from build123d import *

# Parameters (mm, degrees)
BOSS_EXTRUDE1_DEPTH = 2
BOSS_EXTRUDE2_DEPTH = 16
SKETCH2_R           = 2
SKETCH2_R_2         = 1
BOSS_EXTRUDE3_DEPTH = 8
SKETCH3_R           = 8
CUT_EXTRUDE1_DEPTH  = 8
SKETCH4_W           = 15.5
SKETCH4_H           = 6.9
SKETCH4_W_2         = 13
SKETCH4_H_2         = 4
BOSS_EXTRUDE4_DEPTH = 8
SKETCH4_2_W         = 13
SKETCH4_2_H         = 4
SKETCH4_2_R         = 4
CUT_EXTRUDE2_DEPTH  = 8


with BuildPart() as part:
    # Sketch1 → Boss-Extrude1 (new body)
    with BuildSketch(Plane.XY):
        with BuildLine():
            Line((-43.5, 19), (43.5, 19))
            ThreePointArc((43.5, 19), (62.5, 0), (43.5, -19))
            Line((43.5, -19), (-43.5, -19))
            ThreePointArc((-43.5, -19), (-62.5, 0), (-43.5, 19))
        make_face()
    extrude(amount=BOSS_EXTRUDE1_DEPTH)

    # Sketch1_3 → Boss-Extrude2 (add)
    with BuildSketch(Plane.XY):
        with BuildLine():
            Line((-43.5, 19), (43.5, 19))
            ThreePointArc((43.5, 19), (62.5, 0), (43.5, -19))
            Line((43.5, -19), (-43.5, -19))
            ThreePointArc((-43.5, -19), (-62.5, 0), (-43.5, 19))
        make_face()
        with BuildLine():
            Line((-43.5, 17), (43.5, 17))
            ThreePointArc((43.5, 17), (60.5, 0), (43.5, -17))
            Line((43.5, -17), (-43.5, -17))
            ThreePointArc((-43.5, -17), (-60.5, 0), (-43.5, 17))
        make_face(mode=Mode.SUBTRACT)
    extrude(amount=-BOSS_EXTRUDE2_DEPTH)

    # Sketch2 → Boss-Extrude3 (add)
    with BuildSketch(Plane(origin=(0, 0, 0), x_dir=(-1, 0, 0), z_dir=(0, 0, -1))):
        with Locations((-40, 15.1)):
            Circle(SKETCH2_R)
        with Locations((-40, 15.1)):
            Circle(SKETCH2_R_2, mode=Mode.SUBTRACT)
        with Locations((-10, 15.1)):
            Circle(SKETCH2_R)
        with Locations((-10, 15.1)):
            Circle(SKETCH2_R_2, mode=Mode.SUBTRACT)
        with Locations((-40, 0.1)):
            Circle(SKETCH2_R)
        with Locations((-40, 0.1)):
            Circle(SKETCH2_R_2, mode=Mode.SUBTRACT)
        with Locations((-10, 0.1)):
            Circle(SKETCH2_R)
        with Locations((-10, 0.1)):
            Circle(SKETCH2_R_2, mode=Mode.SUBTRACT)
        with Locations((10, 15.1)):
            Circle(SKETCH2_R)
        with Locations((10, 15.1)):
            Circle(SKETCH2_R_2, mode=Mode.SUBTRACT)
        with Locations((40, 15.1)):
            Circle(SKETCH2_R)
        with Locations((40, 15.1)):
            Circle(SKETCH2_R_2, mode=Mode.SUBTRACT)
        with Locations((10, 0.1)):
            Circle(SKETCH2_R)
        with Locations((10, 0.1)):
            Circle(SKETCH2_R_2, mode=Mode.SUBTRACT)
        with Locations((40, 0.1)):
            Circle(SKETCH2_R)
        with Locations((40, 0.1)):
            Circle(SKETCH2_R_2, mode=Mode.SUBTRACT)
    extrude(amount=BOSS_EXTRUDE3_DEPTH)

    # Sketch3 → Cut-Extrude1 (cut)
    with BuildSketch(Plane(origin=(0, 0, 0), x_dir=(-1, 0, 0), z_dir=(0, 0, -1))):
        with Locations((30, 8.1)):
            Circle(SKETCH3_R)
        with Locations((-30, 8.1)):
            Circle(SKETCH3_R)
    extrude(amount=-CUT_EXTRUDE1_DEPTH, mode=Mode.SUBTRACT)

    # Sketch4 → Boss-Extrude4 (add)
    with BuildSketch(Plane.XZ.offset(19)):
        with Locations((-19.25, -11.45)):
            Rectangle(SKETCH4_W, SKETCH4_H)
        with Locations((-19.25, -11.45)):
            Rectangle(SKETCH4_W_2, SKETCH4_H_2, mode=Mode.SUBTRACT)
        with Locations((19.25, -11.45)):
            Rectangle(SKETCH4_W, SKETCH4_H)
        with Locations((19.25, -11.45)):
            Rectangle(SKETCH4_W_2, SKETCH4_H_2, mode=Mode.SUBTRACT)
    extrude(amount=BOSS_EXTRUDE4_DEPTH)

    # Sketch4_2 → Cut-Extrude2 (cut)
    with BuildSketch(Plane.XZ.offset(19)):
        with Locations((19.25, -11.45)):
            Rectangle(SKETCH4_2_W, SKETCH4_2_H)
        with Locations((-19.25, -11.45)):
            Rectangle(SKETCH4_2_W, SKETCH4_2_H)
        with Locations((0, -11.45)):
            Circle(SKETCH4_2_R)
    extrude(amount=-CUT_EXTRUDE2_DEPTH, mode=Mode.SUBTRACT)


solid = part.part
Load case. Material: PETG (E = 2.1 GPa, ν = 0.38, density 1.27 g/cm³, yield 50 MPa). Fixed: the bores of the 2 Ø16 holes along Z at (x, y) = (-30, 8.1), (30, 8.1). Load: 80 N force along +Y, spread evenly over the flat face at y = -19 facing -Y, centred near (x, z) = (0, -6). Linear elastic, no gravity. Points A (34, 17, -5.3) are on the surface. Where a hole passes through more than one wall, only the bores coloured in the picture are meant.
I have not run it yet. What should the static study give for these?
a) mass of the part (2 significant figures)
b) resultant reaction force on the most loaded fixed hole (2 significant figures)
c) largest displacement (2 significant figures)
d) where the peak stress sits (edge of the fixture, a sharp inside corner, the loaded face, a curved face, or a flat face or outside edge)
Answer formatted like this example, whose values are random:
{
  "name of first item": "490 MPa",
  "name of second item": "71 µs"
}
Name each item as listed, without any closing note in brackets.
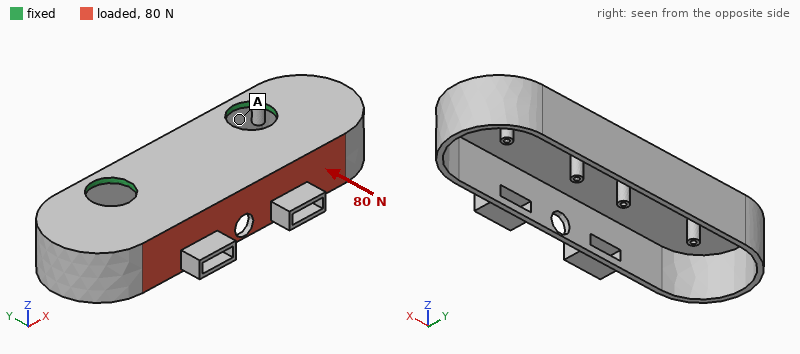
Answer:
{
  "mass of the part": "23 g",
  "resultant reaction force on the most loaded fixed hole": "40 N",
  "largest displacement": "1.3 mm",
  "where the peak stress sits": "a flat face or outside edge"
}
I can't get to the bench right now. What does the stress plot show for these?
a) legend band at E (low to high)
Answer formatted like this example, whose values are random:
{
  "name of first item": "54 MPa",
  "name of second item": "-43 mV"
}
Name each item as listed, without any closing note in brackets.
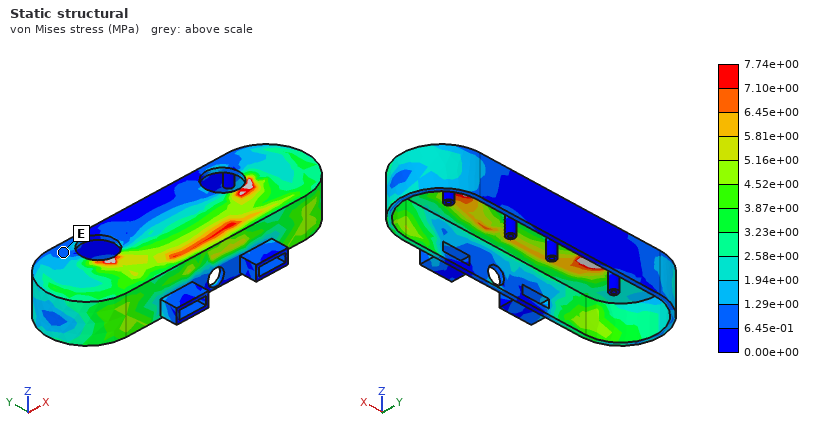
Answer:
{
  "legend band at E": "6.45e-01 to 1.29e+00 MPa"
}
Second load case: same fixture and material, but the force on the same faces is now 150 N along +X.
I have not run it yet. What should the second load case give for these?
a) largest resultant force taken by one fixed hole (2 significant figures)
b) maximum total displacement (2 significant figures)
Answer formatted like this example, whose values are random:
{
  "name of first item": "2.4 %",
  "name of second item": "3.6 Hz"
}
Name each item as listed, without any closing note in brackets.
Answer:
{
  "largest resultant force taken by one fixed hole": "89 N",
  "maximum total displacement": "0.55 mm"
}
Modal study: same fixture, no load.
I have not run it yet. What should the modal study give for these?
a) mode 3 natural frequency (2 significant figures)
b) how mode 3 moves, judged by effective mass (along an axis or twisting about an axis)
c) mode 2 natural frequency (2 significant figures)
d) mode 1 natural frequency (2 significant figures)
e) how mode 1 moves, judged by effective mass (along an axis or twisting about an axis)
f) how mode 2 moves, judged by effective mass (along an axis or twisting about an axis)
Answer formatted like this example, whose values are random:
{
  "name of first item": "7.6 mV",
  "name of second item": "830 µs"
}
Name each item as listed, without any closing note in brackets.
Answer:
{
  "mode 3 natural frequency": "1000 Hz",
  "how mode 3 moves, judged by effective mass": "along Z",
  "mode 2 natural frequency": "480 Hz",
  "mode 1 natural frequency": "400 Hz",
  "how mode 1 moves, judged by effective mass": "along Z",
  "how mode 2 moves, judged by effective mass": "twisting about Y"
}
